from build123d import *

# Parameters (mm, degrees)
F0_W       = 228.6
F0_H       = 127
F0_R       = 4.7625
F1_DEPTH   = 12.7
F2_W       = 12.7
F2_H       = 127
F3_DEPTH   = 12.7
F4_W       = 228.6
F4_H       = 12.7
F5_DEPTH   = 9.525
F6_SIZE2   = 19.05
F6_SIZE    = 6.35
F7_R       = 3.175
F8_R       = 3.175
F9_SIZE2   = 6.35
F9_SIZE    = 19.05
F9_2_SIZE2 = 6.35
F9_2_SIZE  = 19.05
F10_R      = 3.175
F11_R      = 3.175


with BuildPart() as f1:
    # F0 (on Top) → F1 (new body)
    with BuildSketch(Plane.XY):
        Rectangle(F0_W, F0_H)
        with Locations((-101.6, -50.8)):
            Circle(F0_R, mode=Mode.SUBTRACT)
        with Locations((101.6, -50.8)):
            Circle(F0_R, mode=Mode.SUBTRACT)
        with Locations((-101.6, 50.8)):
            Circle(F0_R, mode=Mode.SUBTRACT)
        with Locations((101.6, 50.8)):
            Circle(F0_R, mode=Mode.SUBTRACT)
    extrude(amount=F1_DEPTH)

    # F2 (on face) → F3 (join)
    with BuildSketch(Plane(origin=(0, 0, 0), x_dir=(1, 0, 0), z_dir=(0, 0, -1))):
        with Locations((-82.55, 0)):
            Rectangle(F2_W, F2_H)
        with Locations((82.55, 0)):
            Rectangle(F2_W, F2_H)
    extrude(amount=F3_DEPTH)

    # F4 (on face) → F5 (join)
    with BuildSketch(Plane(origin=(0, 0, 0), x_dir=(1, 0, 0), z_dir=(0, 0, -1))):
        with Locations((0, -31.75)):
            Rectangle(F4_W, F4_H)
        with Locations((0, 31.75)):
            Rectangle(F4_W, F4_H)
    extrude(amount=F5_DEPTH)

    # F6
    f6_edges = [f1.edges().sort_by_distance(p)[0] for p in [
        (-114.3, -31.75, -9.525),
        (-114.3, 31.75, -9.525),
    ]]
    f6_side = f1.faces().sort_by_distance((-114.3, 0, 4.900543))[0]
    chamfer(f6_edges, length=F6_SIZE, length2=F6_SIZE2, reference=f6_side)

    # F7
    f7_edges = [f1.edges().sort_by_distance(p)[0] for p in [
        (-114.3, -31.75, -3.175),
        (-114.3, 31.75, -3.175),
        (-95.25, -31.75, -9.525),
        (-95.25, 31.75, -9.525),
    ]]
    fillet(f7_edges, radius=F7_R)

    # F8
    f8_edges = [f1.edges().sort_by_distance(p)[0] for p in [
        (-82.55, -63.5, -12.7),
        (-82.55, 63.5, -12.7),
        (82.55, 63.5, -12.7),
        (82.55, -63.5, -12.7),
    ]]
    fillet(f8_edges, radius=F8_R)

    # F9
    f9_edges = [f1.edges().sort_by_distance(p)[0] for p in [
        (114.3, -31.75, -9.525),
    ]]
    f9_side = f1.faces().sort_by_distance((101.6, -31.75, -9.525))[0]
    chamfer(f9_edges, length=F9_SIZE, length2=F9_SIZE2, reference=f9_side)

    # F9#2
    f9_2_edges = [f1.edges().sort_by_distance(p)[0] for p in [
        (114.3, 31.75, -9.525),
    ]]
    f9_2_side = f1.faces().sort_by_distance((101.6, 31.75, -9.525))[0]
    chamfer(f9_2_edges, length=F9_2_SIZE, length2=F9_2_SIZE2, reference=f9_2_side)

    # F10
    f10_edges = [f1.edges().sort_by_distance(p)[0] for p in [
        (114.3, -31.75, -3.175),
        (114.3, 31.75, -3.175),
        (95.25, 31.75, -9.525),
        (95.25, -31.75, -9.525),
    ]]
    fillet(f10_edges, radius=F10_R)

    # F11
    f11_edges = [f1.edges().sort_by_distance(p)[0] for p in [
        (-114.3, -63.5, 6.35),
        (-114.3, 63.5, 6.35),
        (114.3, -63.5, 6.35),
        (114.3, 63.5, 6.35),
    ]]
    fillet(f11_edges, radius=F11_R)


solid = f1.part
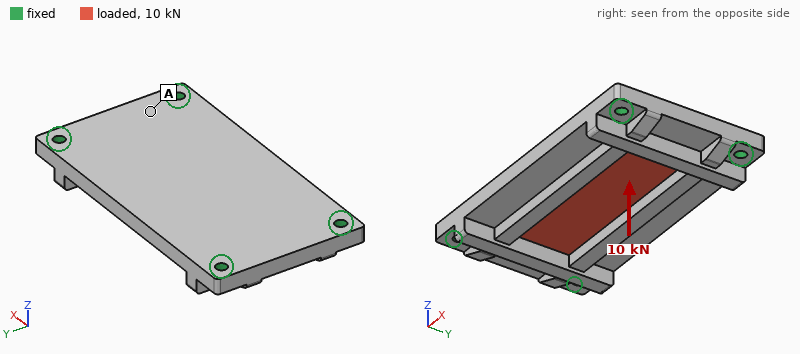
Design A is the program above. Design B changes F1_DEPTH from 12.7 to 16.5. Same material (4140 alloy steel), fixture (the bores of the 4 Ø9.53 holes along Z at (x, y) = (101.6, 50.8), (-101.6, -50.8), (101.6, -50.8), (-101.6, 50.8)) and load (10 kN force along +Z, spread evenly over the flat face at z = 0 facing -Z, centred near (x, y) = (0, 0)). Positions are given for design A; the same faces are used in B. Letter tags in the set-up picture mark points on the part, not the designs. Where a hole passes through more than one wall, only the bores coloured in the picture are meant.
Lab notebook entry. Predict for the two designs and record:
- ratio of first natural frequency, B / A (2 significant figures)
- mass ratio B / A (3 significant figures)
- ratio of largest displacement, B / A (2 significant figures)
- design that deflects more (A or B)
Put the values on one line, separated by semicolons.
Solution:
1.2; 1.24; 0.56; A
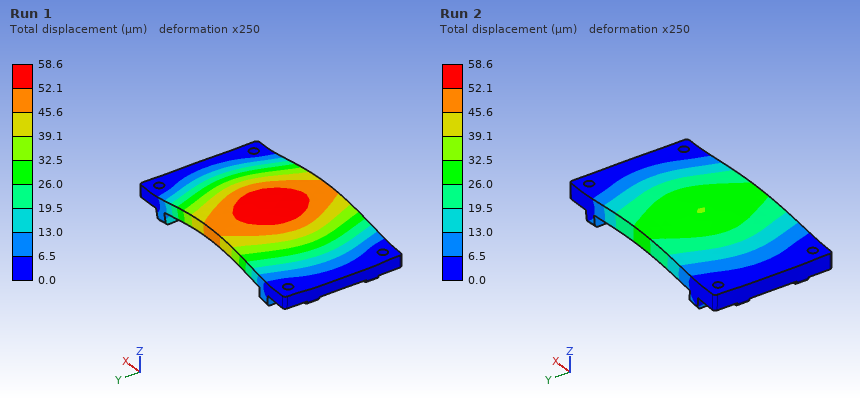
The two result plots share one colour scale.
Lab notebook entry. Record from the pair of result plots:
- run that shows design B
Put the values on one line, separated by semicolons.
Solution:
Run 2
